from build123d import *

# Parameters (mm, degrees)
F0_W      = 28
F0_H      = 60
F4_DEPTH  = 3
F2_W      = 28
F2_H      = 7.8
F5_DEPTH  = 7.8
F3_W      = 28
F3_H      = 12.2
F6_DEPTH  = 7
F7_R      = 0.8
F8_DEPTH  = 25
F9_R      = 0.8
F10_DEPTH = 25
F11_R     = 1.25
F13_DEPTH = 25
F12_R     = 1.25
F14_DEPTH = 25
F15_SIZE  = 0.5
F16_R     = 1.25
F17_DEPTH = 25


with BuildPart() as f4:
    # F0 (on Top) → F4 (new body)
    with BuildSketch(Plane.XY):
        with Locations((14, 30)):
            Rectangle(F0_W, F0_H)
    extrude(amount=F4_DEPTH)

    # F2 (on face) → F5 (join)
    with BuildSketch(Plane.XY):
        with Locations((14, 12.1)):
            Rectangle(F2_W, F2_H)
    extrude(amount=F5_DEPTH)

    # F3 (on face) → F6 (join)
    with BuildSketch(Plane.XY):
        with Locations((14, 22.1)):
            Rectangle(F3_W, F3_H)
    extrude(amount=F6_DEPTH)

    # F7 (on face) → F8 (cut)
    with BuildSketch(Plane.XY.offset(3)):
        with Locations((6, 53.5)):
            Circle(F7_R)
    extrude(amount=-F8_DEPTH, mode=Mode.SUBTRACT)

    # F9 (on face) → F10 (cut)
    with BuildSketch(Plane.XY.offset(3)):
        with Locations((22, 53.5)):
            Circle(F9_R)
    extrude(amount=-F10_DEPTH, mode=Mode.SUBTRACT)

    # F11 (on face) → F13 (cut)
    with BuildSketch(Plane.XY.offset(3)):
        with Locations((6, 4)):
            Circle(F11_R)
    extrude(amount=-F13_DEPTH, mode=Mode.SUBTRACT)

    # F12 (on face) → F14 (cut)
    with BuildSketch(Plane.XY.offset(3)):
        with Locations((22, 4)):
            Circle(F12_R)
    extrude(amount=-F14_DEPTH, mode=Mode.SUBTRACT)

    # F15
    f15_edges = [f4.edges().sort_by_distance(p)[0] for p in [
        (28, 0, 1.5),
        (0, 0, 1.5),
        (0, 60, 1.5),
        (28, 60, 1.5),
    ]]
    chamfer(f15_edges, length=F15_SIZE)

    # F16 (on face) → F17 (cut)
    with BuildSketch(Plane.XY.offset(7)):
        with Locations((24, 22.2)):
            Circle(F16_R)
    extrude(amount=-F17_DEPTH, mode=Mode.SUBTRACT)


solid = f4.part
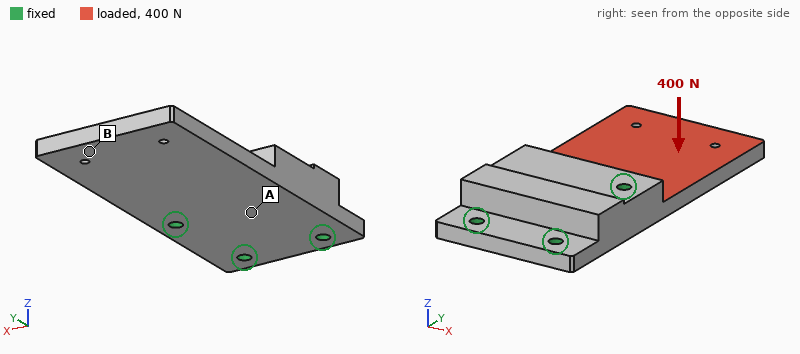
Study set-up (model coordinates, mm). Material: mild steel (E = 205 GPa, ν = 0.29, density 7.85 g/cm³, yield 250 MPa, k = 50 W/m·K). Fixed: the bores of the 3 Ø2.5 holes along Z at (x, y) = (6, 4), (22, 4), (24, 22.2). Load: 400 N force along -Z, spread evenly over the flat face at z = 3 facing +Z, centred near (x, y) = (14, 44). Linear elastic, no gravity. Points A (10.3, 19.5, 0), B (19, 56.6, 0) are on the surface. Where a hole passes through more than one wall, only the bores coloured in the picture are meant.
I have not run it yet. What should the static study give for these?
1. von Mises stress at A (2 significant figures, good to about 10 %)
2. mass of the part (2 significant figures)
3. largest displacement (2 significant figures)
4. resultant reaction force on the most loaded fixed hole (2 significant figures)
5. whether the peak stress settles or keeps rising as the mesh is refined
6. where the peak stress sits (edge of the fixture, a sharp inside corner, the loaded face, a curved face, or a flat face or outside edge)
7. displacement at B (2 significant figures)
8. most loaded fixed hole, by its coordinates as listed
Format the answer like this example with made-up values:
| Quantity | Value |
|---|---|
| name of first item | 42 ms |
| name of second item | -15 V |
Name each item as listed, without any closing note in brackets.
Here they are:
| Quantity | Value |
|---|---|
| von Mises stress at A | 26 MPa |
| mass of the part | 58 g |
| largest displacement | 0.17 mm |
| resultant reaction force on the most loaded fixed hole | 630 N |
| whether the peak stress settles or keeps rising as the mesh is refined | keeps rising |
| where the peak stress sits | edge of the fixture |
| displacement at B | 0.14 mm |
| most loaded fixed hole, by its coordinates as listed | (24, 22.2) |
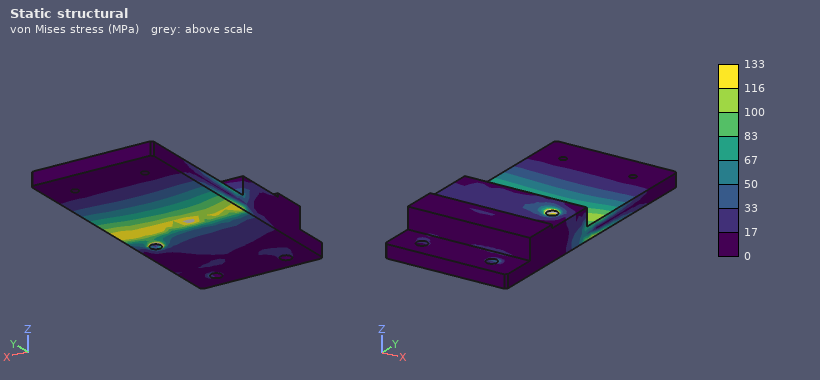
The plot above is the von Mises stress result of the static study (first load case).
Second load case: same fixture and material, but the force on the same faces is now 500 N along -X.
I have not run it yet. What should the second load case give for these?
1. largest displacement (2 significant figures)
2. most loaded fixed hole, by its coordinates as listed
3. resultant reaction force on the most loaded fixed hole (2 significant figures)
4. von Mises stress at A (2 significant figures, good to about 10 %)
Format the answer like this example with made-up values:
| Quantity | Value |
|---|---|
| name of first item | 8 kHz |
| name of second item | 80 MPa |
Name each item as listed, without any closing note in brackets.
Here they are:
| Quantity | Value |
|---|---|
| largest displacement | 12 µm |
| most loaded fixed hole, by its coordinates as listed | (24, 22.2) |
| resultant reaction force on the most loaded fixed hole | 800 N |
| von Mises stress at A | 9.0 MPa |
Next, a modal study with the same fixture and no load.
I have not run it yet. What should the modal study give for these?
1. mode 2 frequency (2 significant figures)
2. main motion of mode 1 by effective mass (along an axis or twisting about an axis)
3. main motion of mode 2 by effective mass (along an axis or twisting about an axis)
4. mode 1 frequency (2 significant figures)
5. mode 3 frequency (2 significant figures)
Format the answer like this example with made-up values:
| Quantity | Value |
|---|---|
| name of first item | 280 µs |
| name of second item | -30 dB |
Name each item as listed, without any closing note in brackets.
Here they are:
| Quantity | Value |
|---|---|
| mode 2 frequency | 5600 Hz |
| main motion of mode 1 by effective mass | along Z |
| main motion of mode 2 by effective mass | twisting about Y |
| mode 1 frequency | 2100 Hz |
| mode 3 frequency | 9500 Hz |
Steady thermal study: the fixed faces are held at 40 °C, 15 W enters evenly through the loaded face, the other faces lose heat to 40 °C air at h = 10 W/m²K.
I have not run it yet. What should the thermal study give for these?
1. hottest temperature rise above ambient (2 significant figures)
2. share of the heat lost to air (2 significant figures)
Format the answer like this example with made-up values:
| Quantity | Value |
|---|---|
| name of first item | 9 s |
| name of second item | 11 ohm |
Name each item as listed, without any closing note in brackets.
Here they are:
| Quantity | Value |
|---|---|
| hottest temperature rise above ambient | 77 K |
| share of the heat lost to air | 6.0 % |
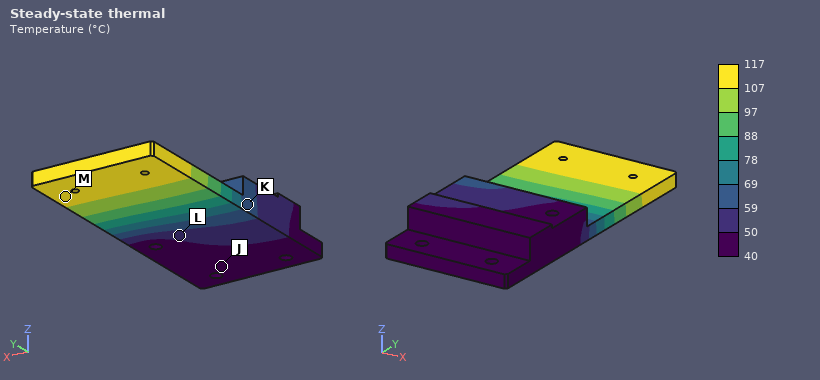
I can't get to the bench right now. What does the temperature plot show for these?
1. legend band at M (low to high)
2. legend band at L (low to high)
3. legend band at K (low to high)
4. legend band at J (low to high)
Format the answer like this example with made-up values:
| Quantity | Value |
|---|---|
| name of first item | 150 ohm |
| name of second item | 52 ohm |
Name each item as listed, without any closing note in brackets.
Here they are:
| Quantity | Value |
|---|---|
| legend band at M | 107 to 117 °C |
| legend band at L | 50 to 59 °C |
| legend band at K | 59 to 69 °C |
| legend band at J | 40 to 50 °C |
